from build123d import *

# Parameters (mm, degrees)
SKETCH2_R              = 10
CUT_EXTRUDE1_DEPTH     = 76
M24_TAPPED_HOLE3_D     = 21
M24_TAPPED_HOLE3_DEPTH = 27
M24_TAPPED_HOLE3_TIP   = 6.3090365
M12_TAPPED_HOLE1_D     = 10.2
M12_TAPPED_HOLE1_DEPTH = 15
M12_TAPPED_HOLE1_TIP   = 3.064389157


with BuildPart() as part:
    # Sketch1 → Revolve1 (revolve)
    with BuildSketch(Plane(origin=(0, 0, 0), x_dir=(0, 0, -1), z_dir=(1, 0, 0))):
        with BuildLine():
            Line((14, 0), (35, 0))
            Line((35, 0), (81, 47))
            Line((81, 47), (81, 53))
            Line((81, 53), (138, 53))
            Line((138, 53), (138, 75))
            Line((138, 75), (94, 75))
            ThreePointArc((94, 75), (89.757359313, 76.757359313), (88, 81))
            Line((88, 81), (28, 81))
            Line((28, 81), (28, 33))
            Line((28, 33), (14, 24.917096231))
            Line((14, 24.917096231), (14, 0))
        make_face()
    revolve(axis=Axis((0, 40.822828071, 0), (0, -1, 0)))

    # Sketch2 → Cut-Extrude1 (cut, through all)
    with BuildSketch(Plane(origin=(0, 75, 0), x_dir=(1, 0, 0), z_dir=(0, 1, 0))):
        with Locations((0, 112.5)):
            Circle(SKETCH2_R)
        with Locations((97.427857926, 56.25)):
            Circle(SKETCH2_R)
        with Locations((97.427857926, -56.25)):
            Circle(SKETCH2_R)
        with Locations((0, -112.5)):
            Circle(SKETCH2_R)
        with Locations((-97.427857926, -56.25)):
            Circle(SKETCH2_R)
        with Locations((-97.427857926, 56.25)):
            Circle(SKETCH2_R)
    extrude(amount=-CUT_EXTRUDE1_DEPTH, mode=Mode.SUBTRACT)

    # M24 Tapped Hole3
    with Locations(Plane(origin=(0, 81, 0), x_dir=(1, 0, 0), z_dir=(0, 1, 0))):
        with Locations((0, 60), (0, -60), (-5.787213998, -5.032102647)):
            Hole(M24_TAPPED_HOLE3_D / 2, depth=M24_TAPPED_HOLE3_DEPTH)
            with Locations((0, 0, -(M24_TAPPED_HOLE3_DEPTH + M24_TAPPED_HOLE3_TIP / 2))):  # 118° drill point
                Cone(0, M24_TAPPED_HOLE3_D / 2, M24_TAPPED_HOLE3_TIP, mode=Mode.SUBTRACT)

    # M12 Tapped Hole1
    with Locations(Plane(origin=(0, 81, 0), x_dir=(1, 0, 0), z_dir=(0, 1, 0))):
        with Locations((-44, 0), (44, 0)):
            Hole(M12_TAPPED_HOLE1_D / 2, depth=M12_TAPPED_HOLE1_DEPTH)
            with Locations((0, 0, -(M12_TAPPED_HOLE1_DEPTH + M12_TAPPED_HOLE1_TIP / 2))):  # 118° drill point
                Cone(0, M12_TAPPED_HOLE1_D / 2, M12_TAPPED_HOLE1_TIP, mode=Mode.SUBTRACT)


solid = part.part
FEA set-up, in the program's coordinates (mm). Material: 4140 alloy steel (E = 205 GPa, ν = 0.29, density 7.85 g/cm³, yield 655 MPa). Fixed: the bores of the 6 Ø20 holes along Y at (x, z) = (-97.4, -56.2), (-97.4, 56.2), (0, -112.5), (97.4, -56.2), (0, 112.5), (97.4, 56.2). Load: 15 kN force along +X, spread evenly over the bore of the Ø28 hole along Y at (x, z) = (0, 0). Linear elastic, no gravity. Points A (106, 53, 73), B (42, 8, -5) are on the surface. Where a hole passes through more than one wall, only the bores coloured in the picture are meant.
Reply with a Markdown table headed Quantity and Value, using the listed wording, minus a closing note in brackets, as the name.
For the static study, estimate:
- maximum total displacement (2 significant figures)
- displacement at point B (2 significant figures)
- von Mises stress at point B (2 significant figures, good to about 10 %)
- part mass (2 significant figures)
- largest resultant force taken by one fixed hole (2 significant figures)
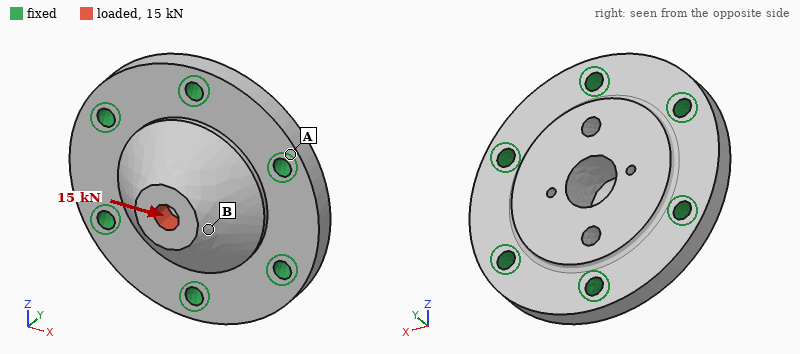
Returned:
| Quantity | Value |
|---|---|
| maximum total displacement | 3.7 µm |
| displacement at point B | 2.9 µm |
| von Mises stress at point B | 4.0 MPa |
| part mass | 15 kg |
| largest resultant force taken by one fixed hole | 3.9 kN |
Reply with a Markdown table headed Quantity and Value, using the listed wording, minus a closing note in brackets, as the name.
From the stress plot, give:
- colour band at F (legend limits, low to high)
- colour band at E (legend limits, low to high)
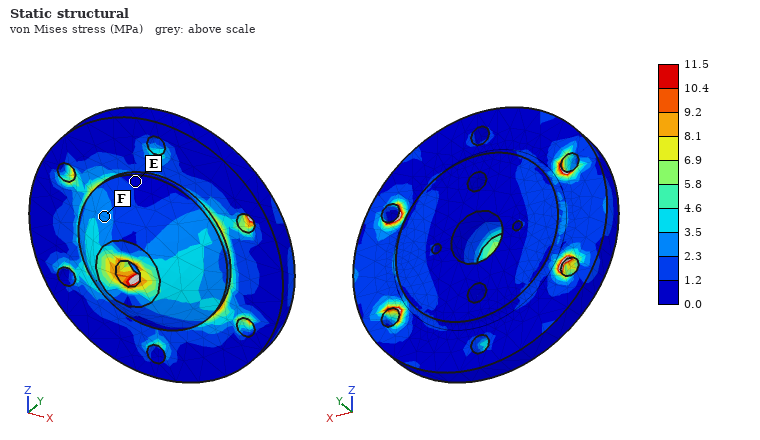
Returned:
| Quantity | Value |
|---|---|
| colour band at F | 2.3 to 3.5 MPa |
| colour band at E | 0.0 to 1.2 MPa |
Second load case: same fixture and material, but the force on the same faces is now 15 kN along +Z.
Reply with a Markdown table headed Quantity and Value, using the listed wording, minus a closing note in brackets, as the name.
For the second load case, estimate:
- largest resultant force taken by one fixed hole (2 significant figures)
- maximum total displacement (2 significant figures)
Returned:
| Quantity | Value |
|---|---|
| largest resultant force taken by one fixed hole | 4.4 kN |
| maximum total displacement | 3.7 µm |
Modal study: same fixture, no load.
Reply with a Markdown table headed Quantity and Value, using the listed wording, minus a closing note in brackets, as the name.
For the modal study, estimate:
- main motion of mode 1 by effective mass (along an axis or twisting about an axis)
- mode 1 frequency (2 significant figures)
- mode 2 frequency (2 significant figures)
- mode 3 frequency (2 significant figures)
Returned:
| Quantity | Value |
|---|---|
| main motion of mode 1 by effective mass | along Y |
| mode 1 frequency | 4400 Hz |
| mode 2 frequency | 6200 Hz |
| mode 3 frequency | 6200 Hz |
